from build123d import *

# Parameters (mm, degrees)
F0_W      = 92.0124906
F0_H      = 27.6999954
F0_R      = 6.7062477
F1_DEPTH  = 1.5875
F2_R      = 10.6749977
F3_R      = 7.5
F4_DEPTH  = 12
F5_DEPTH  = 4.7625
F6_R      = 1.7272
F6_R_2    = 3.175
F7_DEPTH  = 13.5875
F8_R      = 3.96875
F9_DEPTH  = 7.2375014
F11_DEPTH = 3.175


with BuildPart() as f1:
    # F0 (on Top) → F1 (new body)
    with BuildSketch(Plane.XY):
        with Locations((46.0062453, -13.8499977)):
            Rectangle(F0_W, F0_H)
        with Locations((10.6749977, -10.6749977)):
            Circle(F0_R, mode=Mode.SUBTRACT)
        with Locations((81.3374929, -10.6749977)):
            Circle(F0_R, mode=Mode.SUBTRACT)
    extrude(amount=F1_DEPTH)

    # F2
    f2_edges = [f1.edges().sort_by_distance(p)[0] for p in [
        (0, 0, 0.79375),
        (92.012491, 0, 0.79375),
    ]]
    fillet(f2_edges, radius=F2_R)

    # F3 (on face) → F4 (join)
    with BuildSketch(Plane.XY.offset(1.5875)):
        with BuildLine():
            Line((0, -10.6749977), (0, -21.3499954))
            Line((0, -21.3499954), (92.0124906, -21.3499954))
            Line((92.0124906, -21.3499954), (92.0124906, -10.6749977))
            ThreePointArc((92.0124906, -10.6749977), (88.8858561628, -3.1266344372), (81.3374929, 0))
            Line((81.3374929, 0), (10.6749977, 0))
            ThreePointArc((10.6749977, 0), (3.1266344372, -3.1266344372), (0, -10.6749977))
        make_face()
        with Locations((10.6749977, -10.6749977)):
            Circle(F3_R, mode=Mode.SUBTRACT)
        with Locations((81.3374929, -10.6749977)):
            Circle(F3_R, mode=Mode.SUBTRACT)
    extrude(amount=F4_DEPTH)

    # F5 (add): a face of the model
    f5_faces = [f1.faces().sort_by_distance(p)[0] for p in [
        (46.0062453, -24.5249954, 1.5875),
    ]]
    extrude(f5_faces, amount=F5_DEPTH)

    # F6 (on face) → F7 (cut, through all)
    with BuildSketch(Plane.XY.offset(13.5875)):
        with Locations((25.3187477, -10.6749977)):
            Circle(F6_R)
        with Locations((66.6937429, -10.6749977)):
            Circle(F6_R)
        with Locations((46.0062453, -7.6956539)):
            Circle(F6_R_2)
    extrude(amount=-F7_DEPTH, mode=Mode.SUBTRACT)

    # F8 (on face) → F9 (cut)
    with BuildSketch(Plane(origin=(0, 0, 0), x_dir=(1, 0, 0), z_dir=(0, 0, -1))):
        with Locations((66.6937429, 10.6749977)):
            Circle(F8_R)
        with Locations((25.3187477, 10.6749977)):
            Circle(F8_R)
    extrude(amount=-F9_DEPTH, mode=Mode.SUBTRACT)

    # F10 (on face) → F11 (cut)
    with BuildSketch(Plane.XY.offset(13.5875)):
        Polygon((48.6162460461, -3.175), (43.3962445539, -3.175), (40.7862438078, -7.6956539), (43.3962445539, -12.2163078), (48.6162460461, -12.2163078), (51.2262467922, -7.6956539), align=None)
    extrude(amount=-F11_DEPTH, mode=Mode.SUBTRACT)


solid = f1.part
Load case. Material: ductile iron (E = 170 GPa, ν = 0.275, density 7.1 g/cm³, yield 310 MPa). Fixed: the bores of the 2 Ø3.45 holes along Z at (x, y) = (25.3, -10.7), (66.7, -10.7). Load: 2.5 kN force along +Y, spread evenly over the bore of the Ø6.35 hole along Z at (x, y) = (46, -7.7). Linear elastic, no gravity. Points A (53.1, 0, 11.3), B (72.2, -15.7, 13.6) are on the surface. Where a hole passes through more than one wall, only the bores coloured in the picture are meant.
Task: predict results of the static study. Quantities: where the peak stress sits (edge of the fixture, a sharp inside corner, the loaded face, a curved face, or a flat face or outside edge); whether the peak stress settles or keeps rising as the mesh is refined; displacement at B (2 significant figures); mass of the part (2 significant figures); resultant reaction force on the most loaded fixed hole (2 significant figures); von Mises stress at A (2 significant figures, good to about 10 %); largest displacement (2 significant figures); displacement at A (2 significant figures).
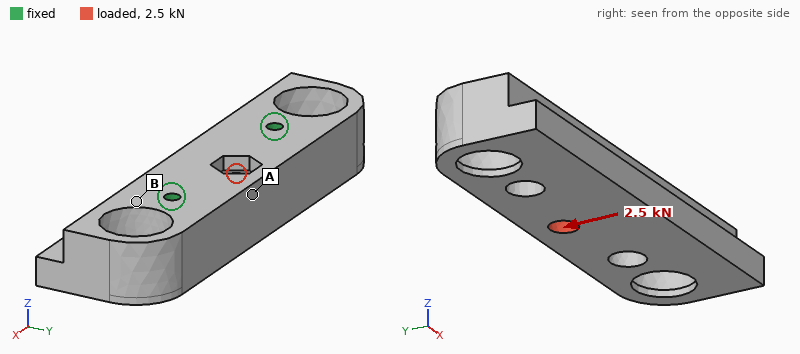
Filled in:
edge of the fixture
keeps rising
1.7 µm
170 g
1.3 kN
14 MPa
8.8 µm
4.1 µm
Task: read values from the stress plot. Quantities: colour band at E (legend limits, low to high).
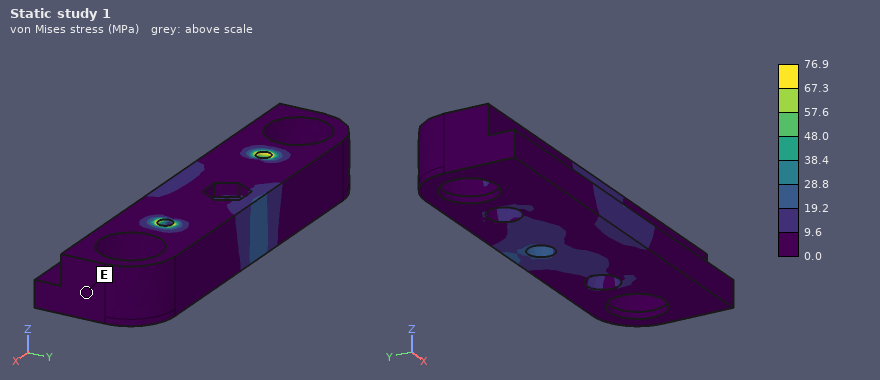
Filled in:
0.0 to 9.6 MPa
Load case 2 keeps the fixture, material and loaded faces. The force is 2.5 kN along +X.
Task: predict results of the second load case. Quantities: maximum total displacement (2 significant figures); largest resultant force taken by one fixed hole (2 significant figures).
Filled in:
1.6 µm
1.3 kN
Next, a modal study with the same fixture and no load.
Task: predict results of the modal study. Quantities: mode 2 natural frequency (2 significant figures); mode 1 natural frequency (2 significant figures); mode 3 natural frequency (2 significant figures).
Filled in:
8700 Hz
7300 Hz
9700 Hz
